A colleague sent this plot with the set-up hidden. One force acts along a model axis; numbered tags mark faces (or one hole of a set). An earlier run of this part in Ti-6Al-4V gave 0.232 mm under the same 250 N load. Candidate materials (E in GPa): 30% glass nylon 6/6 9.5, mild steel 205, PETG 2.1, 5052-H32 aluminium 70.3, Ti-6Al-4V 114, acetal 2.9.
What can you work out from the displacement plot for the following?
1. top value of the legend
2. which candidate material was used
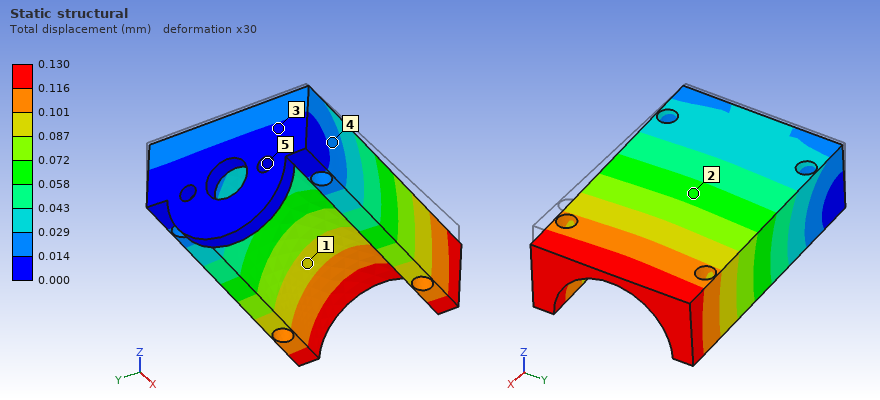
0.130 mm
mild steel
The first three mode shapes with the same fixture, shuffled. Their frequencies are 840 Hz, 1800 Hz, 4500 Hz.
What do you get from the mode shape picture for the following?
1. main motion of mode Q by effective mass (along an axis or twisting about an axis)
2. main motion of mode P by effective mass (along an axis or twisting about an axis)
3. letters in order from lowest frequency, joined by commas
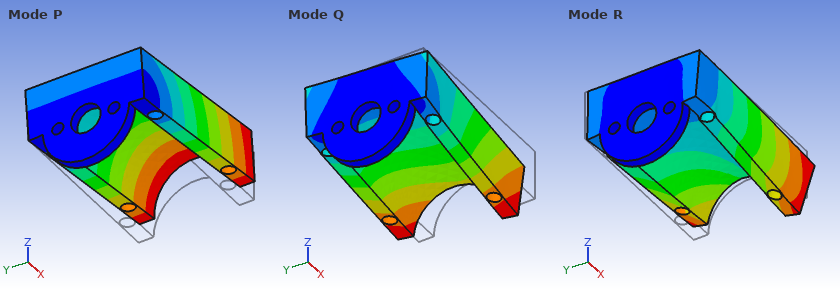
along Y
along Z
P, Q, R
